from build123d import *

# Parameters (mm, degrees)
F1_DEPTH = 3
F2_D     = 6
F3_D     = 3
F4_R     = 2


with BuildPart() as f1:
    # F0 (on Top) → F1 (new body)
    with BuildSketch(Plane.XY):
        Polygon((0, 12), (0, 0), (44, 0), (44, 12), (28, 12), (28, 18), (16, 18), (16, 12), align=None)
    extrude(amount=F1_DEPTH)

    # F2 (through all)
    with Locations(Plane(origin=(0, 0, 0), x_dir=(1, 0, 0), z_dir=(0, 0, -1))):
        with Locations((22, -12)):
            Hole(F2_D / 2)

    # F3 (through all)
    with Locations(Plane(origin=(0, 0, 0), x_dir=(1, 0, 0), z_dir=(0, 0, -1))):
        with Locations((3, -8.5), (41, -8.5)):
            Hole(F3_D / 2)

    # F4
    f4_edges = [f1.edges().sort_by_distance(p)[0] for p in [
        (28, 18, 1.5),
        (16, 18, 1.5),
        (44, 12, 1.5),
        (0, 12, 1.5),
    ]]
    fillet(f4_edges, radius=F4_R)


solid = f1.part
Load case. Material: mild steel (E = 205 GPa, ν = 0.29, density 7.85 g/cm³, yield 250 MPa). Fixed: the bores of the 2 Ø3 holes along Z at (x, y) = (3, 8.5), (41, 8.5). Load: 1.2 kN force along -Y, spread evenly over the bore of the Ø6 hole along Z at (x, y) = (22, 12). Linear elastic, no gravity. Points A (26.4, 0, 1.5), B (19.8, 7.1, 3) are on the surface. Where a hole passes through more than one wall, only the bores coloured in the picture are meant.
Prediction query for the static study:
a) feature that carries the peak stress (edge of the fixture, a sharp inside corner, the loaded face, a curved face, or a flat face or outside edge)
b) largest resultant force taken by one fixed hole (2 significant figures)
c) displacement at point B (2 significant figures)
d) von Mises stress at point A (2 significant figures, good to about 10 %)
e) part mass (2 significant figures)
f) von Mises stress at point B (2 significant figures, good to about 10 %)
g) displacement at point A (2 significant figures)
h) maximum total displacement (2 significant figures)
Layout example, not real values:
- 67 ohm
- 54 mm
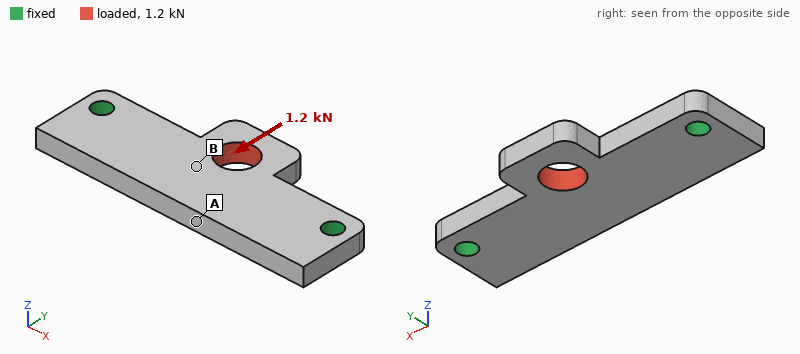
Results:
- edge of the fixture
- 720 N
- 10 µm
- 79 MPa
- 13 g
- 22 MPa
- 9.1 µm
- 11 µm
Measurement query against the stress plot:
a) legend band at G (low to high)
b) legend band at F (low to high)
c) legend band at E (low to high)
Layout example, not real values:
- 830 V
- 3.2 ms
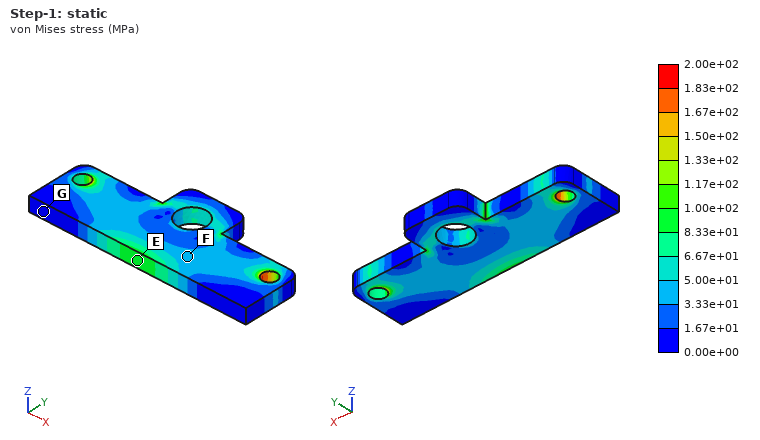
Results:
- 0.00e+00 to 1.67e+01 MPa
- 3.33e+01 to 5.00e+01 MPa
- 8.33e+01 to 1.00e+02 MPa
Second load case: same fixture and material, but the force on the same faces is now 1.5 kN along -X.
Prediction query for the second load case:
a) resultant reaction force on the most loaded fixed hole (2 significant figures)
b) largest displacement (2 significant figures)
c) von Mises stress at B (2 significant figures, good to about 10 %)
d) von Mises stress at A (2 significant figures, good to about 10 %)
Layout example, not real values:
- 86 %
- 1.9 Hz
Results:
- 770 N
- 7.6 µm
- 17 MPa
- 11 MPa
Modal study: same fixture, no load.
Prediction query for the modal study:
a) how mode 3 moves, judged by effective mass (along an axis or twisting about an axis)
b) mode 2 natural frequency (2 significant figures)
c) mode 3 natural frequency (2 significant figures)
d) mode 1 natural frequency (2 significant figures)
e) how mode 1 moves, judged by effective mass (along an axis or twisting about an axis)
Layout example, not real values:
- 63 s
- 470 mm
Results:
- along Y
- 12 kHz
- 21 kHz
- 9100 Hz
- along Z
